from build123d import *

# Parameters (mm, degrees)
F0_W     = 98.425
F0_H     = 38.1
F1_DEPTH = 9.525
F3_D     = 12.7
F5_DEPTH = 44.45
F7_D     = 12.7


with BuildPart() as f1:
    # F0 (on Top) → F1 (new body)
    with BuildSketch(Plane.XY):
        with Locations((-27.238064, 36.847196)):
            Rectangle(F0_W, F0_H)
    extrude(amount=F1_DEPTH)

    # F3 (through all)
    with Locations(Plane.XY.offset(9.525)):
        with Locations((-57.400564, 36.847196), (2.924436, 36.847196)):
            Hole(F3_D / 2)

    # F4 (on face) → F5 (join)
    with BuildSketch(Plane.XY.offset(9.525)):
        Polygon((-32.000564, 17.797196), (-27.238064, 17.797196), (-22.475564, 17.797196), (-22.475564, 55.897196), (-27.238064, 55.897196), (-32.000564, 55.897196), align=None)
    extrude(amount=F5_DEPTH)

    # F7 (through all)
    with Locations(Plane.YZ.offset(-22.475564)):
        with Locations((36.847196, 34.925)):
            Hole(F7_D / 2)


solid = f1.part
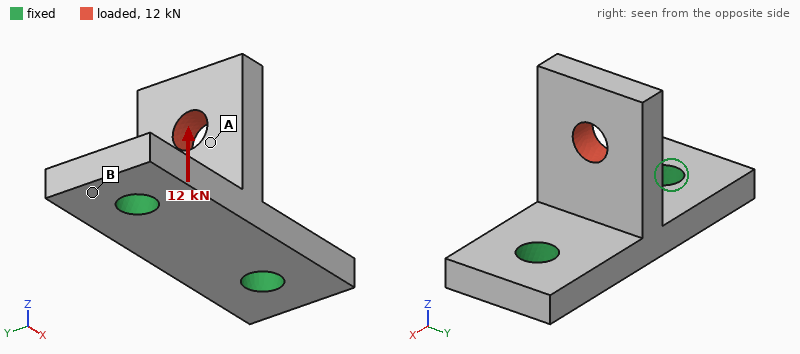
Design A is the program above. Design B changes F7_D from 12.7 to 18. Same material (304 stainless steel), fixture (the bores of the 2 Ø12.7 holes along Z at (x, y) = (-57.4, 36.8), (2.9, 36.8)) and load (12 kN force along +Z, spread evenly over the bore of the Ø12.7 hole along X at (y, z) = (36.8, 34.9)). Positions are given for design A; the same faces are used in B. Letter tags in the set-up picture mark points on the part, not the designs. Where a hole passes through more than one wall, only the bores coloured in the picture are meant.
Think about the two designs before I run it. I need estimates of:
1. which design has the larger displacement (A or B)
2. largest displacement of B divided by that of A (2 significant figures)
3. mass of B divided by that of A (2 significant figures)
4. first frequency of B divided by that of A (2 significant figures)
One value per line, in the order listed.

B
1.1
0.97
1.0
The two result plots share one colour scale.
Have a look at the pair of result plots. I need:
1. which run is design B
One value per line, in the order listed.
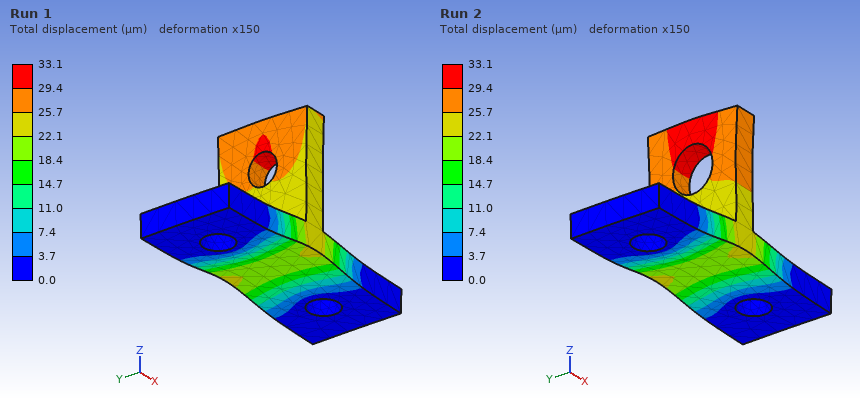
Run 2
